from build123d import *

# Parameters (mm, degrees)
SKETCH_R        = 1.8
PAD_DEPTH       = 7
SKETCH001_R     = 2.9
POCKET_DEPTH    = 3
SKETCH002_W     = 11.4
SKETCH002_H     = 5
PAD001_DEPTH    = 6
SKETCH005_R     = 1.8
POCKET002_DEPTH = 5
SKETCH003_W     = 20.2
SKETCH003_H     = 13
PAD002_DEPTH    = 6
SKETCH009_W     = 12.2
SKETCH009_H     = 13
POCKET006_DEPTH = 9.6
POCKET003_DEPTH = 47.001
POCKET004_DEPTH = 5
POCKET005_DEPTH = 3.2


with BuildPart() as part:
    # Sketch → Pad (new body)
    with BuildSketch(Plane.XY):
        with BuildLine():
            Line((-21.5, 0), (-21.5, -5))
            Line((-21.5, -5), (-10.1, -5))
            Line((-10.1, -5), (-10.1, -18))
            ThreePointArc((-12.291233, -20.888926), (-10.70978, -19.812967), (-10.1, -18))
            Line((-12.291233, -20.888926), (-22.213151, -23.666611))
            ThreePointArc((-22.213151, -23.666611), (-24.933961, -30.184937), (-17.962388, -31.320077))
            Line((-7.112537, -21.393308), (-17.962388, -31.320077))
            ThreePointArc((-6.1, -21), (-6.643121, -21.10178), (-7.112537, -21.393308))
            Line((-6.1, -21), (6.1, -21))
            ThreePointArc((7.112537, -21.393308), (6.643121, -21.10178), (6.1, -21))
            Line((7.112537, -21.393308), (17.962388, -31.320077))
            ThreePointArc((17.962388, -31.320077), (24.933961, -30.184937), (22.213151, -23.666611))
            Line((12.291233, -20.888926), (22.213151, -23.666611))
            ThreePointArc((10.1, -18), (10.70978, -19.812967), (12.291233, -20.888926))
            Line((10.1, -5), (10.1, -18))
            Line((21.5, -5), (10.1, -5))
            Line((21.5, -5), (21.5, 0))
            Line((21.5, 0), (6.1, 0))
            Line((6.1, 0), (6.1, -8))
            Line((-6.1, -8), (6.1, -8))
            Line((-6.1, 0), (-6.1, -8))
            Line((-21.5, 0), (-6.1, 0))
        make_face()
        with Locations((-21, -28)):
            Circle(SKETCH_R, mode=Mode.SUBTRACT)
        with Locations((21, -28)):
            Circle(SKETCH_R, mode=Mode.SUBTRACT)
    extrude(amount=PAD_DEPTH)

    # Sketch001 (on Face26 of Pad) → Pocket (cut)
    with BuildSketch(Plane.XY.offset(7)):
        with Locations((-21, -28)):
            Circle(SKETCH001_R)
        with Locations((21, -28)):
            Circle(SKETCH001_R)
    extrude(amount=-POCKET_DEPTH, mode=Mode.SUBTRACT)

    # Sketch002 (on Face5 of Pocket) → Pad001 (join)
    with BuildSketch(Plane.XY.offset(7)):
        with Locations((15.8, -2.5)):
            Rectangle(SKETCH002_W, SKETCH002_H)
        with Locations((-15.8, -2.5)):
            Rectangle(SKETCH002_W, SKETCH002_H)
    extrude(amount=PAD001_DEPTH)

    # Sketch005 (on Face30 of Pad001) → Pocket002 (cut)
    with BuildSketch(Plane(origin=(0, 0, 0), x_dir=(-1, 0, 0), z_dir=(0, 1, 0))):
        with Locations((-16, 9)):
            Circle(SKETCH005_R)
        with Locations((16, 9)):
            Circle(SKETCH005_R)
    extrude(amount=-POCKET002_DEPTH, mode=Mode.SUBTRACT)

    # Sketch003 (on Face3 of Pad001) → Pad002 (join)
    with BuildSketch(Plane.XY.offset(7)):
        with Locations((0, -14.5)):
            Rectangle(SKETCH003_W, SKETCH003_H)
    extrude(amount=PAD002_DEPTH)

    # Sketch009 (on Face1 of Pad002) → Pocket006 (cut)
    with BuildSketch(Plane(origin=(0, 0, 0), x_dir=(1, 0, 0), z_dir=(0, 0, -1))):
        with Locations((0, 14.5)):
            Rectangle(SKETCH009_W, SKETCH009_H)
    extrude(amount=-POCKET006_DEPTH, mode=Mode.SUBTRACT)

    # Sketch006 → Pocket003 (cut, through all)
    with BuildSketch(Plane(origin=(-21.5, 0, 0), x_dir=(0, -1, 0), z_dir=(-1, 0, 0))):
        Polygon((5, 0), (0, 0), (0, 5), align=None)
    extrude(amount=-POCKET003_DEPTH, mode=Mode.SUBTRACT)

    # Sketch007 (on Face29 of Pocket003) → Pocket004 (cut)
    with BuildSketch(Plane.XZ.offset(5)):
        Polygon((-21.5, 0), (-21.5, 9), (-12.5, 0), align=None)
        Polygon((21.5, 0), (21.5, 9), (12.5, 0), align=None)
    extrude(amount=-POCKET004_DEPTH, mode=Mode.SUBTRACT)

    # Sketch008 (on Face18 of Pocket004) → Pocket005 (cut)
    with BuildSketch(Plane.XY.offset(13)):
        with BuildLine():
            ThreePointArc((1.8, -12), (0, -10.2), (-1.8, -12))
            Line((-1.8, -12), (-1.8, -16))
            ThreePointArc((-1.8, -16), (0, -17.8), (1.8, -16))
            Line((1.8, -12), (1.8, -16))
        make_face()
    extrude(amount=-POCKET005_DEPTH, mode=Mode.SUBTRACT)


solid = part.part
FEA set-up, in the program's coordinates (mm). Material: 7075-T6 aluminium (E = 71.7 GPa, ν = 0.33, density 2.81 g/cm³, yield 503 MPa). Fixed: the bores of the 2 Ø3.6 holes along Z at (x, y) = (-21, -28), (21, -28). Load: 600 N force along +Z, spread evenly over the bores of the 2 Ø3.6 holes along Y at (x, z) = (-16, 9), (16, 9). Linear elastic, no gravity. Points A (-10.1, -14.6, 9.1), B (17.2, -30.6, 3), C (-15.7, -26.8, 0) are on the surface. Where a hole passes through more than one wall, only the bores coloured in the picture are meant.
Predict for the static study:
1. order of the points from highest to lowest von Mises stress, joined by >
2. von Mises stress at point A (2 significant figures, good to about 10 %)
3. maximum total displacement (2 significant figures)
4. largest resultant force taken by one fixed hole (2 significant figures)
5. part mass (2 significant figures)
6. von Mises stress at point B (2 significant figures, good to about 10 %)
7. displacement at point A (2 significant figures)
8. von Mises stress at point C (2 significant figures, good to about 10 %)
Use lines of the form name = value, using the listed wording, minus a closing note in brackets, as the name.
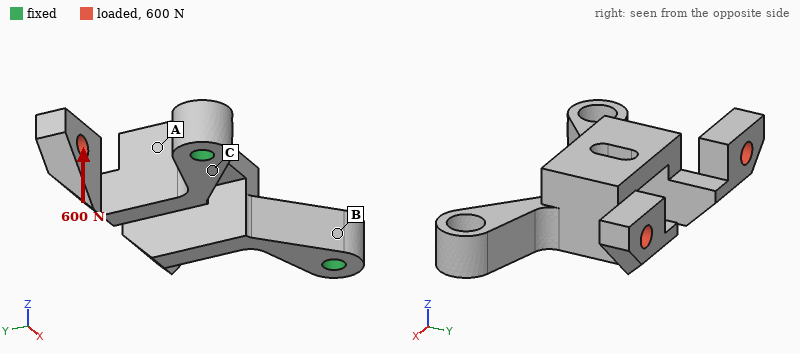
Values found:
order of the points from highest to lowest von Mises stress, joined by > = C > B > A
von Mises stress at point A = 49 MPa
maximum total displacement = 0.68 mm
largest resultant force taken by one fixed hole = 330 N
part mass = 12 g
von Mises stress at point B = 120 MPa
displacement at point A = 0.22 mm
von Mises stress at point C = 180 MPa
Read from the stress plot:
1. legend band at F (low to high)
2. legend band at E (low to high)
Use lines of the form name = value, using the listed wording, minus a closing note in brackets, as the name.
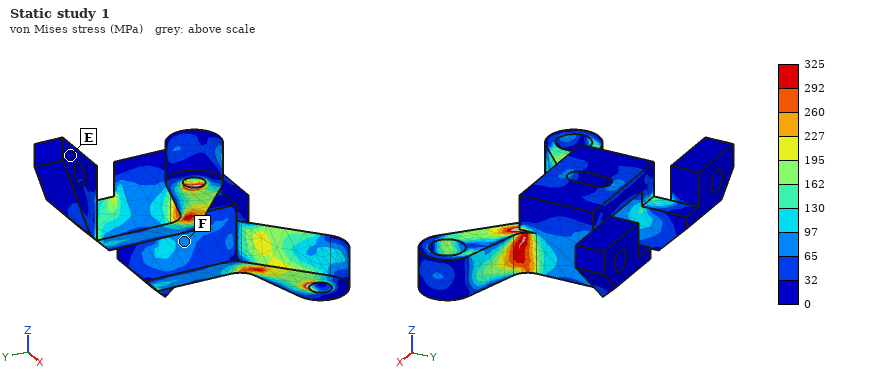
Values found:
legend band at F = 65 to 97 MPa
legend band at E = 0 to 32 MPa
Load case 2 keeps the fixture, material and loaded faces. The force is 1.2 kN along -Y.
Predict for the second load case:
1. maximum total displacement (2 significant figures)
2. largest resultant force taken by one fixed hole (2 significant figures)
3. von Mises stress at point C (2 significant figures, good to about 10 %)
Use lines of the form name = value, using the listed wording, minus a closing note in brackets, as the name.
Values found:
maximum total displacement = 0.60 mm
largest resultant force taken by one fixed hole = 620 N
von Mises stress at point C = 52 MPa
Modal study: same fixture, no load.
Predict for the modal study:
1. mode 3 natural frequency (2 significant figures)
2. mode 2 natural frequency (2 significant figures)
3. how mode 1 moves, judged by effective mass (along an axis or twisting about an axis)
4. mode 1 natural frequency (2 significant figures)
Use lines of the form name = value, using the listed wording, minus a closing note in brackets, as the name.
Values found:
mode 3 natural frequency = 5600 Hz
mode 2 natural frequency = 3800 Hz
how mode 1 moves, judged by effective mass = along Z
mode 1 natural frequency = 2600 Hz
